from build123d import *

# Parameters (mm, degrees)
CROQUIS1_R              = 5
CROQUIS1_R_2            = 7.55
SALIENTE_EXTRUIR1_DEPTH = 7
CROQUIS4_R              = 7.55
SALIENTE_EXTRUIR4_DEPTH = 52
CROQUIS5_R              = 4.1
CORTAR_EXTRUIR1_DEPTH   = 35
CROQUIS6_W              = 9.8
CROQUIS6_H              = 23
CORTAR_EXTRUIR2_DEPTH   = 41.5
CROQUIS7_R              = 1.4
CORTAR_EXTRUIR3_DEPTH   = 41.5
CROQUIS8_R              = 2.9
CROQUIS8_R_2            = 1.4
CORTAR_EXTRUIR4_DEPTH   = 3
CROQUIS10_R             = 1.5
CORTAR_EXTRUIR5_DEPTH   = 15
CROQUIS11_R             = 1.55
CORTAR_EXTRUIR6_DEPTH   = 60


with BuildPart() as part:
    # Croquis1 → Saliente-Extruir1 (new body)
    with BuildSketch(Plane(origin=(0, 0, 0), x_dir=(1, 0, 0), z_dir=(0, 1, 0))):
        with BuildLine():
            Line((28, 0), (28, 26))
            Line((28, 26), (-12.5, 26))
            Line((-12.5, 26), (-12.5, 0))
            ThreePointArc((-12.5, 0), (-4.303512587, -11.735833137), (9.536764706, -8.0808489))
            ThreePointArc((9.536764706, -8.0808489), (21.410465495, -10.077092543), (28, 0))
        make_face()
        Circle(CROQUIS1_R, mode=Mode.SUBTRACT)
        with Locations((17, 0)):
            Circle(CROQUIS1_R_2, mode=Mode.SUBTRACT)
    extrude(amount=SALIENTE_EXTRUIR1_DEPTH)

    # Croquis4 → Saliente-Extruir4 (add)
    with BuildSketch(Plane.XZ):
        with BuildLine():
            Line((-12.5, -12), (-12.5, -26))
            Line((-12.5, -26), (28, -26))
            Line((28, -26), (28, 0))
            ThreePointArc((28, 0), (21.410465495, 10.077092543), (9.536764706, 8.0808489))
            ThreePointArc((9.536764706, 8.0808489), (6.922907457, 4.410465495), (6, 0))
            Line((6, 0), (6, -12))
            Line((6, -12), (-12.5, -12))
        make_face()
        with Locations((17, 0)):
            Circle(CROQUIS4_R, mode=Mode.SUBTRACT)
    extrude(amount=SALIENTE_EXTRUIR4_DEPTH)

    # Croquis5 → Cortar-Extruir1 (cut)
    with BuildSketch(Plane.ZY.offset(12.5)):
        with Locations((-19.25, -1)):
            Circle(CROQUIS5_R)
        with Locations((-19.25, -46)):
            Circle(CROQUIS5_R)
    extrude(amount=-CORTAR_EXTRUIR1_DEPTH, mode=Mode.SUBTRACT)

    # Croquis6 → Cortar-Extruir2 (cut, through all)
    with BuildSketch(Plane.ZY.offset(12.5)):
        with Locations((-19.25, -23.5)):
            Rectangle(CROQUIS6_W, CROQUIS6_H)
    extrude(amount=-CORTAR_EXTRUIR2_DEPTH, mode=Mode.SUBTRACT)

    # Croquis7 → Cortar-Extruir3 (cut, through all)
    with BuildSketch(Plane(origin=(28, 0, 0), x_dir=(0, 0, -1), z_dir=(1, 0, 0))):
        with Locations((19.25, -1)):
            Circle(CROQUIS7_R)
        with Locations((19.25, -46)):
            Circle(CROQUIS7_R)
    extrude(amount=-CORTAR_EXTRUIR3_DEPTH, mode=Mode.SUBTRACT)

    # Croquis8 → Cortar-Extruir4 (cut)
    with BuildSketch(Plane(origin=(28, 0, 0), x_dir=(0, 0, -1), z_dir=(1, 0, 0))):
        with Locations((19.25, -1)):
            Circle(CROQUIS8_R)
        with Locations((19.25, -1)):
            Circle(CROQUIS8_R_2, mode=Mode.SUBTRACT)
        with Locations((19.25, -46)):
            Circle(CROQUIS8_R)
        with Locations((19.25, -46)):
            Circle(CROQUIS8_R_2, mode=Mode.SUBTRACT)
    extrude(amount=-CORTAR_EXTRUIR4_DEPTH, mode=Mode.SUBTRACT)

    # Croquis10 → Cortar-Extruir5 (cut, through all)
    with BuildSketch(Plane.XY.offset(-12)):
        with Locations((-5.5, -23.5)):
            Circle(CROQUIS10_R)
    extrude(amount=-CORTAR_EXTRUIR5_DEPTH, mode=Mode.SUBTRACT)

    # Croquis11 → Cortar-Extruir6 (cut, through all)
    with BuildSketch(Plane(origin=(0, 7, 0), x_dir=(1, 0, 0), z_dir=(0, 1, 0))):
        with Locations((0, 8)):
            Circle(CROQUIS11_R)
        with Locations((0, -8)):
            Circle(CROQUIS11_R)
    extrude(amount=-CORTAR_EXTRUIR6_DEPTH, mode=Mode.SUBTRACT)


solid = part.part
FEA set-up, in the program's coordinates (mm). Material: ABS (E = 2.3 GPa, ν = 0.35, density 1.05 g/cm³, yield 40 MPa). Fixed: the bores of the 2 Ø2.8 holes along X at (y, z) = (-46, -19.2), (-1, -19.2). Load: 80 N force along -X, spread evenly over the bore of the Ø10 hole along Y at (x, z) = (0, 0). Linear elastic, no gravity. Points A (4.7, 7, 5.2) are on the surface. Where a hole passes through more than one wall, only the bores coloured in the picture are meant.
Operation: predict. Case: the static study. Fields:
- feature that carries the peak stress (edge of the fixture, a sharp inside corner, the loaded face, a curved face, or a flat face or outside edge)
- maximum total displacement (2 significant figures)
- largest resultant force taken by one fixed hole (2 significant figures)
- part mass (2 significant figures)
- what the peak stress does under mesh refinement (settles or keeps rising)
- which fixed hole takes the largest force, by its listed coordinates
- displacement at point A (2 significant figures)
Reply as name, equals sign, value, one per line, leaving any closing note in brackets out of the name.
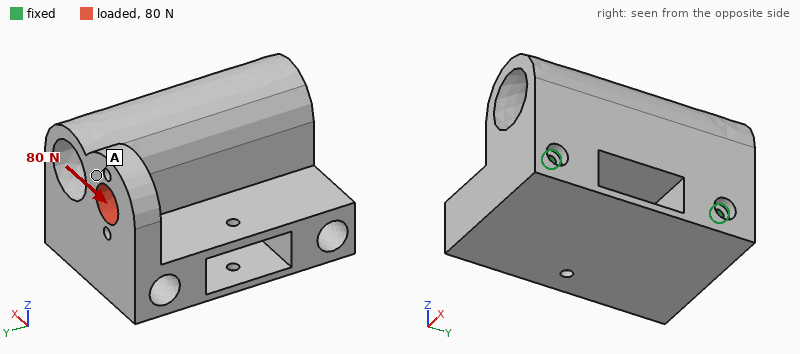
feature that carries the peak stress = edge of the fixture
maximum total displacement = 0.90 mm
largest resultant force taken by one fixed hole = 87 N
part mass = 41 g
what the peak stress does under mesh refinement = keeps rising
which fixed hole takes the largest force, by its listed coordinates = (-1, -19.2)
displacement at point A = 0.66 mm
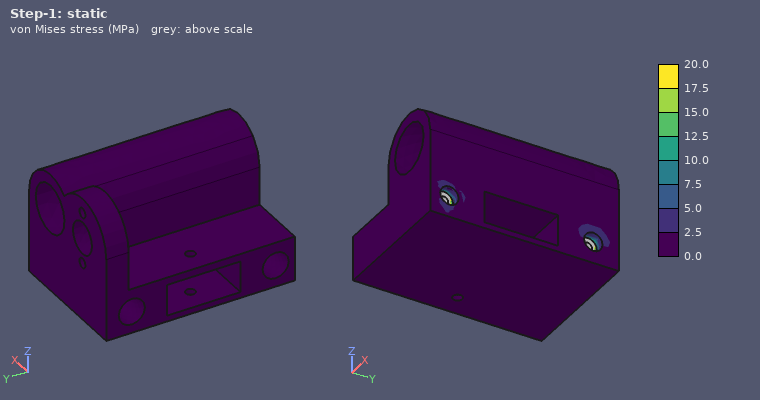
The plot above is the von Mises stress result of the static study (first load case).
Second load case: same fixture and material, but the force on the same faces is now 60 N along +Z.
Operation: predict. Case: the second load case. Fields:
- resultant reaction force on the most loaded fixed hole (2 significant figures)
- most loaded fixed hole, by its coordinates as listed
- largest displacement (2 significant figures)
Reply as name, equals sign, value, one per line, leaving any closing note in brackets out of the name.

resultant reaction force on the most loaded fixed hole = 65 N
most loaded fixed hole, by its coordinates as listed = (-1, -19.2)
largest displacement = 0.83 mm
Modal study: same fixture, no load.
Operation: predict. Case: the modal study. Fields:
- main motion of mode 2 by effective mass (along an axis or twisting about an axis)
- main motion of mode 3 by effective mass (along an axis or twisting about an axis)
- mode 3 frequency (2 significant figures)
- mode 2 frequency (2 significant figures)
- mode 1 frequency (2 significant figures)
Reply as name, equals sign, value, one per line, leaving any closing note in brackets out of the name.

main motion of mode 2 by effective mass = along Y
main motion of mode 3 by effective mass = along Y
mode 3 frequency = 2300 Hz
mode 2 frequency = 2000 Hz
mode 1 frequency = 320 Hz
